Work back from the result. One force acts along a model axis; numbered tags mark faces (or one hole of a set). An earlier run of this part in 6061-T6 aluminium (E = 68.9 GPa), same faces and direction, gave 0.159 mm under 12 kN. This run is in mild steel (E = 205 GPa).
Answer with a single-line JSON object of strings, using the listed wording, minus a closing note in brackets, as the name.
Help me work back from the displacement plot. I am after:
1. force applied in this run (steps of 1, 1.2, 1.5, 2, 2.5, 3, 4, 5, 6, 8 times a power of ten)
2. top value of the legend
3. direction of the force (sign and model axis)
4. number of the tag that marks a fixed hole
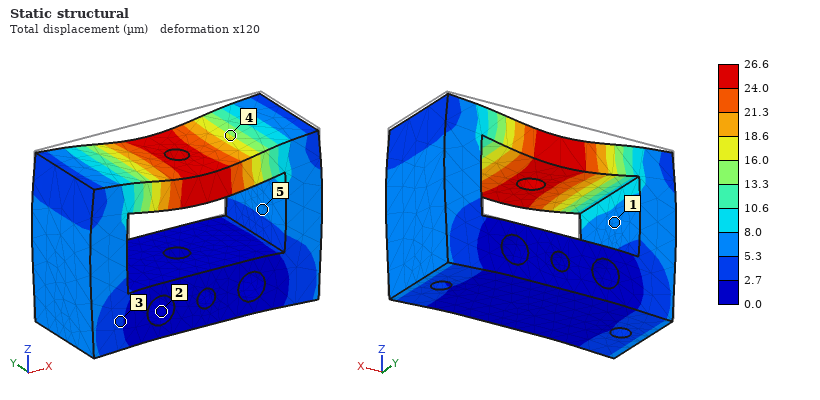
{"force applied in this run": "6 kN", "top value of the legend": "26.6 µm", "direction of the force": "-Z", "number of the tag that marks a fixed hole": "2"}
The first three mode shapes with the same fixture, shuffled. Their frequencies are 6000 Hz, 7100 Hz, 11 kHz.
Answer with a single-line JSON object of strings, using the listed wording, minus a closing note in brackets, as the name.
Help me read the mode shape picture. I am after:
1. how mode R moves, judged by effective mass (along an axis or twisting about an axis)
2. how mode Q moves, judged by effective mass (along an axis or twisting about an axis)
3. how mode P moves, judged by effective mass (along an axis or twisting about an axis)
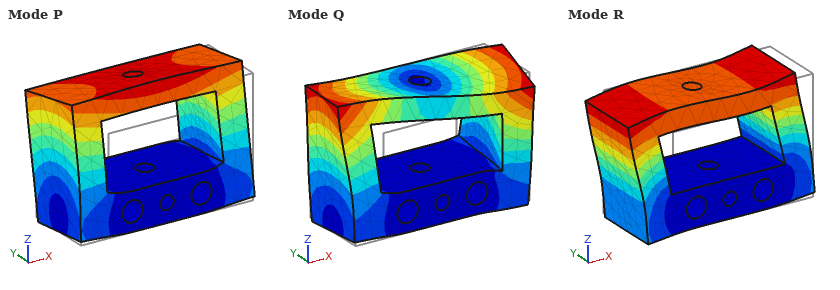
{"how mode R moves, judged by effective mass": "along X", "how mode Q moves, judged by effective mass": "twisting about Z", "how mode P moves, judged by effective mass": "along Y"}
